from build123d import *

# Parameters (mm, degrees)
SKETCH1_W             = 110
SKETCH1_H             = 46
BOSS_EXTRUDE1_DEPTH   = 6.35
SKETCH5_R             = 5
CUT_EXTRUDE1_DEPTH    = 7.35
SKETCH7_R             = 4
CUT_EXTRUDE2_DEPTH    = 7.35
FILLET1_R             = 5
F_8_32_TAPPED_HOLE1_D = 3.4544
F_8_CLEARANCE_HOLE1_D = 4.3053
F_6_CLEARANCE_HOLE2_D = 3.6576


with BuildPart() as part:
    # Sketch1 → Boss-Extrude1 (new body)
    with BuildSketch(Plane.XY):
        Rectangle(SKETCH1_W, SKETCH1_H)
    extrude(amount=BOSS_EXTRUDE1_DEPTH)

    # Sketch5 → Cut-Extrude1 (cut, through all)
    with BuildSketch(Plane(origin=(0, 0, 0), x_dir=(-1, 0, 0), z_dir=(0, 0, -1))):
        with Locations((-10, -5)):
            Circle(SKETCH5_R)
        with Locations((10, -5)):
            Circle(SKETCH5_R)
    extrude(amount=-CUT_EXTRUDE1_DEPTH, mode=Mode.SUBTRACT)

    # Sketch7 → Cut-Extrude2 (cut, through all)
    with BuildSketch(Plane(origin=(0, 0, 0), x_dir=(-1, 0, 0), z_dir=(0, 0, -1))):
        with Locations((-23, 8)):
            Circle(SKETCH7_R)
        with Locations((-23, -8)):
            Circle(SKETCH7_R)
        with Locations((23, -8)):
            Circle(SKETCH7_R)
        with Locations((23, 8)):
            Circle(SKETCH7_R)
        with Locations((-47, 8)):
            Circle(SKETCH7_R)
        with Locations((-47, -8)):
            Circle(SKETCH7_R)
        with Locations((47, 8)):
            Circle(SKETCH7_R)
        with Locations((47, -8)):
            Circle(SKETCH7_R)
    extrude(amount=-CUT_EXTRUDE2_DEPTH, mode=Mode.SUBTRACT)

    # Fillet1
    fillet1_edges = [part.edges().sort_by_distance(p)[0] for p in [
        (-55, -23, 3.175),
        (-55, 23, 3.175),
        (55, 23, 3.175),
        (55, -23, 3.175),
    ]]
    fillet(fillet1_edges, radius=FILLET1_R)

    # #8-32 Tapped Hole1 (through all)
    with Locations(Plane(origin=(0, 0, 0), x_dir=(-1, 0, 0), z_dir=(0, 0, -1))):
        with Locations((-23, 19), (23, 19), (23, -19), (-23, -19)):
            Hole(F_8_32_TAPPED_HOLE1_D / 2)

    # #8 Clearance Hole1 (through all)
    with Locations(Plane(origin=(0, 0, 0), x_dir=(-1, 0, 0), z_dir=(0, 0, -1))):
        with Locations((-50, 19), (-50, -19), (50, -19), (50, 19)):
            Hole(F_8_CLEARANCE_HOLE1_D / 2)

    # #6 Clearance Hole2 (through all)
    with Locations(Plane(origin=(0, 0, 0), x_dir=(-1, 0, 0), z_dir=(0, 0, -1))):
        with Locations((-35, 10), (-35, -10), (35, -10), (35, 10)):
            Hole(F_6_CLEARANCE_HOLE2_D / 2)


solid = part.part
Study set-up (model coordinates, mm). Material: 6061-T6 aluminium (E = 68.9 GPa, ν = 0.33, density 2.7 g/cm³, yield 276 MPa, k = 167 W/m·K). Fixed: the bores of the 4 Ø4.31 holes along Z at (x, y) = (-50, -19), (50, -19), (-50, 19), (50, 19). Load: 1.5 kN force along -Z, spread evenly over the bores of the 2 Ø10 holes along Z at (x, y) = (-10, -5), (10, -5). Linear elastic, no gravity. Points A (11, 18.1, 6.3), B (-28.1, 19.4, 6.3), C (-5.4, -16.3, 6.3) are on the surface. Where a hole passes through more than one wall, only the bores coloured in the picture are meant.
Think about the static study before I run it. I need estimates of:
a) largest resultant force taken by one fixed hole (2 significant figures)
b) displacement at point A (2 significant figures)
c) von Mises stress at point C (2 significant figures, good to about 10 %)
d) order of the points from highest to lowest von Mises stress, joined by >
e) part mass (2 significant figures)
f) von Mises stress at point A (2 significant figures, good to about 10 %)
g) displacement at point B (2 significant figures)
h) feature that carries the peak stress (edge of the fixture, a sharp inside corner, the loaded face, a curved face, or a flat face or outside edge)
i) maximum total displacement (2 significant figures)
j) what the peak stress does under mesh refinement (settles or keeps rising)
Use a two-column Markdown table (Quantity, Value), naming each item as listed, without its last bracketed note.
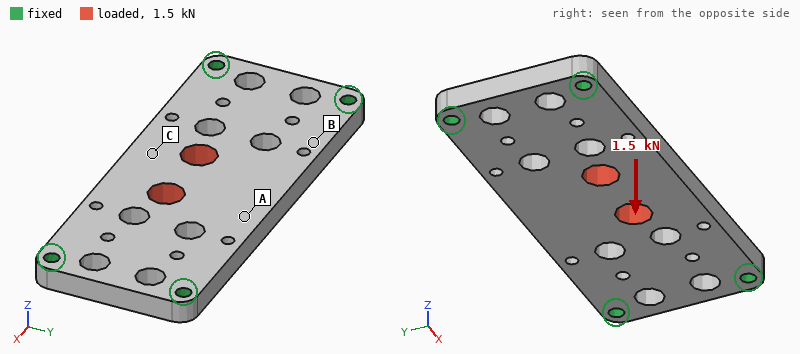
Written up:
| Quantity | Value |
|---|---|
| largest resultant force taken by one fixed hole | 470 N |
| displacement at point A | 0.11 mm |
| von Mises stress at point C | 54 MPa |
| order of the points from highest to lowest von Mises stress, joined by > | C > A > B |
| part mass | 74 g |
| von Mises stress at point A | 33 MPa |
| displacement at point B | 0.055 mm |
| feature that carries the peak stress | edge of the fixture |
| maximum total displacement | 0.17 mm |
| what the peak stress does under mesh refinement | keeps rising |
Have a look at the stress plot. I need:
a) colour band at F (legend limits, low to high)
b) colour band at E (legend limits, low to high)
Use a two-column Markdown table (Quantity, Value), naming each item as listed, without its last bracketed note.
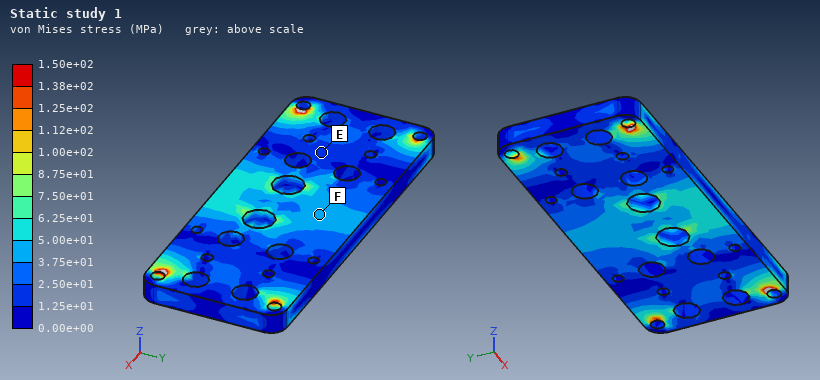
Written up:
| Quantity | Value |
|---|---|
| colour band at F | 3.75e+01 to 5.00e+01 MPa |
| colour band at E | 1.25e+01 to 2.50e+01 MPa |
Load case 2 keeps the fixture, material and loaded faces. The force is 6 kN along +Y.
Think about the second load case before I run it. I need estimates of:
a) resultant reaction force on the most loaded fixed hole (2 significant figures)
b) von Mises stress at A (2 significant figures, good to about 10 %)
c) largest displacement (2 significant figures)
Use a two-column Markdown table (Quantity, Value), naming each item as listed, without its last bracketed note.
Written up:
| Quantity | Value |
|---|---|
| resultant reaction force on the most loaded fixed hole | 2.4 kN |
| von Mises stress at A | 15 MPa |
| largest displacement | 42 µm |
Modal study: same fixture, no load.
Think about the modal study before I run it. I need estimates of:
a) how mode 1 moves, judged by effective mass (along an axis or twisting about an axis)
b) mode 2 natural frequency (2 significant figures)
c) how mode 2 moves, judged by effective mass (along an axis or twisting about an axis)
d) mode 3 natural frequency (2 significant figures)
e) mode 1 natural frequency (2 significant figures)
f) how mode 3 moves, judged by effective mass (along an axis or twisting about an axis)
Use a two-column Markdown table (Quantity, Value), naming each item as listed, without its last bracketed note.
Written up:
| Quantity | Value |
|---|---|
| how mode 1 moves, judged by effective mass | along Z |
| mode 2 natural frequency | 5100 Hz |
| how mode 2 moves, judged by effective mass | twisting about X |
| mode 3 natural frequency | 7600 Hz |
| mode 1 natural frequency | 2900 Hz |
| how mode 3 moves, judged by effective mass | twisting about Y |
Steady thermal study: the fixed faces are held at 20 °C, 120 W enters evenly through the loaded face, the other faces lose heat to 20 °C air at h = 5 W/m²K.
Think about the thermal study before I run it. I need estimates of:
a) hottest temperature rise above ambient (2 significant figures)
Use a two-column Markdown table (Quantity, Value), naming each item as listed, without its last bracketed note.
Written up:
| Quantity | Value |
|---|---|
| hottest temperature rise above ambient | 81 K |
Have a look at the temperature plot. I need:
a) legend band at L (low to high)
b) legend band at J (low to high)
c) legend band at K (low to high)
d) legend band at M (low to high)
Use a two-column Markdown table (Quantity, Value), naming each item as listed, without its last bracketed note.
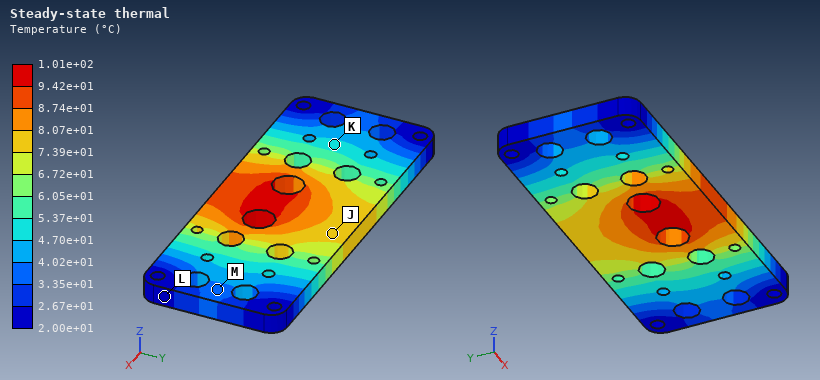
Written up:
| Quantity | Value |
|---|---|
| legend band at L | 2.00e+01 to 2.67e+01 °C |
| legend band at J | 7.39e+01 to 8.07e+01 °C |
| legend band at K | 4.70e+01 to 5.37e+01 °C |
| legend band at M | 3.35e+01 to 4.02e+01 °C |
